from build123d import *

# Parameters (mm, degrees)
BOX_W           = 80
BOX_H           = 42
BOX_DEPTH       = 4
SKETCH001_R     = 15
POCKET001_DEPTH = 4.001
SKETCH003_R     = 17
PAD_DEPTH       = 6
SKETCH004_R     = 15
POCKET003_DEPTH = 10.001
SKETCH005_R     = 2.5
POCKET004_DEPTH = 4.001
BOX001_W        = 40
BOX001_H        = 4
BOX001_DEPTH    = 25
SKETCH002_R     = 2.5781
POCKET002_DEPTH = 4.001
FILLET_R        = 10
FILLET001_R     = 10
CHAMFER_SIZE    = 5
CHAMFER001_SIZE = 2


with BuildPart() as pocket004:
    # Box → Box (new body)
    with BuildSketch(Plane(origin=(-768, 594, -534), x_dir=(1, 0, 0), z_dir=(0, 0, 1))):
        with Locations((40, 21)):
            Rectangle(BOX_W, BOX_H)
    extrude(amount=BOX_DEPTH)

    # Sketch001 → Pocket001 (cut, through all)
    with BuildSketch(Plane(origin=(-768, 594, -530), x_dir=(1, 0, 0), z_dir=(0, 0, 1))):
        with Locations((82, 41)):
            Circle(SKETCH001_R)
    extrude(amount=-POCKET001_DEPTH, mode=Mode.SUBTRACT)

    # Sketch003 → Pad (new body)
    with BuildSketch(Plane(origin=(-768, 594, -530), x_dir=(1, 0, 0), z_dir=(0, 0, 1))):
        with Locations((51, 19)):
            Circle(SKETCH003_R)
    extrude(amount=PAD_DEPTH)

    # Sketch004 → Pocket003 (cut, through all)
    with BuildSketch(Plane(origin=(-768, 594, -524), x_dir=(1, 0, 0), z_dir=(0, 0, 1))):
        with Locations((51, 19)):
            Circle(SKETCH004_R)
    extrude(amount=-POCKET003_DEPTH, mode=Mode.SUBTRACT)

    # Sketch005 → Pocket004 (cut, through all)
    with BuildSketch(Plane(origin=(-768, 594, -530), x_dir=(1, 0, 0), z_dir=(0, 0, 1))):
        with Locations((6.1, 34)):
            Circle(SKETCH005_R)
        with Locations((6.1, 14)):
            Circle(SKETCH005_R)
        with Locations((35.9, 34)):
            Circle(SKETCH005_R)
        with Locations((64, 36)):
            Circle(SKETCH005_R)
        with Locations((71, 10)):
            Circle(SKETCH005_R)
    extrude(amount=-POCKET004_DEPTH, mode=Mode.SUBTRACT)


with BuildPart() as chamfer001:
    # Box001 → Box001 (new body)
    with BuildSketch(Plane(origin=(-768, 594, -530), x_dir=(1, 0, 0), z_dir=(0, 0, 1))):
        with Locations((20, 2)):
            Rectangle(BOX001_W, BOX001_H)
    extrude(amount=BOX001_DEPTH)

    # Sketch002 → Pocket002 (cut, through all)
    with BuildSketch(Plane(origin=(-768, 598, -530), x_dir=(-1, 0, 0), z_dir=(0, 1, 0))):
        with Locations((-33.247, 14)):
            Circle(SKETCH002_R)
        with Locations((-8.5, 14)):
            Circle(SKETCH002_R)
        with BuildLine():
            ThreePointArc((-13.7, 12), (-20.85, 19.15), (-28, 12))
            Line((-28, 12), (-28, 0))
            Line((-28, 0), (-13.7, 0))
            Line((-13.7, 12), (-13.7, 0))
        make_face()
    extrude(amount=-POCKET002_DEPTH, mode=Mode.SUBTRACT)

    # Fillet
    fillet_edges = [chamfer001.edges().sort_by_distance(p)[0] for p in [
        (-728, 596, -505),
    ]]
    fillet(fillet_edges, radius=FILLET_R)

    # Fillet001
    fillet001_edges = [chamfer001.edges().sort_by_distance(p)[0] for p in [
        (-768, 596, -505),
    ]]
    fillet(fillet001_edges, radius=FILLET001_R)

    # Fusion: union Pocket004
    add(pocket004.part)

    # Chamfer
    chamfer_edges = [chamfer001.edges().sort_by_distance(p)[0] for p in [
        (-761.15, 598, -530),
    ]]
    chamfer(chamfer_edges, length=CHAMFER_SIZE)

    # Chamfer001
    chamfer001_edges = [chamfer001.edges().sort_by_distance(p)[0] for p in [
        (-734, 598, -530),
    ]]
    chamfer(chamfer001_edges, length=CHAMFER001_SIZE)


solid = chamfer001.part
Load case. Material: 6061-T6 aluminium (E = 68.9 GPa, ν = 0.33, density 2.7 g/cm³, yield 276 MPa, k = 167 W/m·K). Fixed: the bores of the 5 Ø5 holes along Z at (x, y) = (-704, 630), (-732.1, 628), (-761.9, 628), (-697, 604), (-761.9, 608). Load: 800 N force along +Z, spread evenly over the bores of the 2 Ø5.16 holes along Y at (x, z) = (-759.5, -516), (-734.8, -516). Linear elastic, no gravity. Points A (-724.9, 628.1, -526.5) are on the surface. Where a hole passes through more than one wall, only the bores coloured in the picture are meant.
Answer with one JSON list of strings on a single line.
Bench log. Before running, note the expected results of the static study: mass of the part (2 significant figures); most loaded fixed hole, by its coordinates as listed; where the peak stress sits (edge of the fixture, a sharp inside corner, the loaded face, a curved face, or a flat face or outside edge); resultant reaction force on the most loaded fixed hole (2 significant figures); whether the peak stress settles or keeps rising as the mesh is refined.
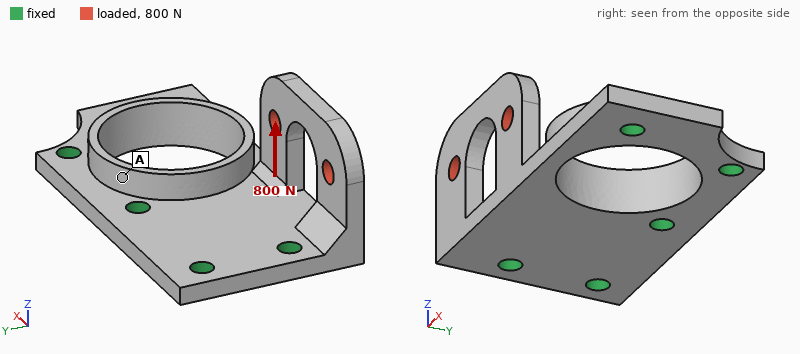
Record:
["37 g", "(-761.9, 608)", "edge of the fixture", "670 N", "keeps rising"]
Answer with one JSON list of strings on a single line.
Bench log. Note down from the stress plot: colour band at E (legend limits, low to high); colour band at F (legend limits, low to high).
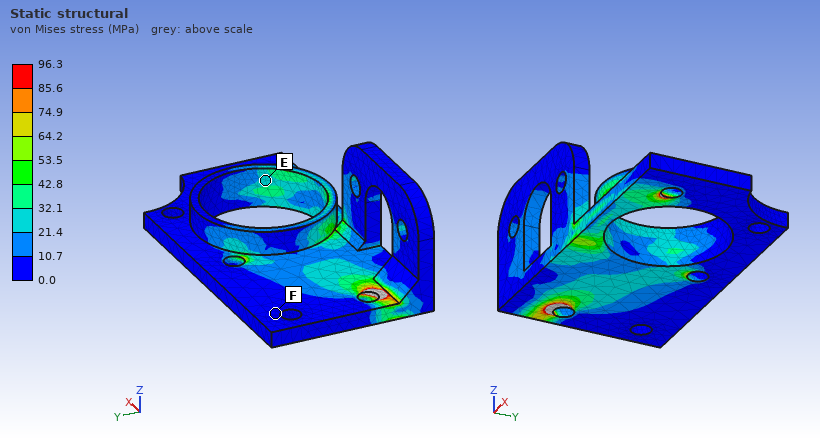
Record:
["21.4 to 32.1 MPa", "0.0 to 10.7 MPa"]
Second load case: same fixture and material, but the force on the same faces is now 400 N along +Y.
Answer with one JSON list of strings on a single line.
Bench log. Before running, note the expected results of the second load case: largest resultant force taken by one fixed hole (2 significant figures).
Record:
["200 N"]
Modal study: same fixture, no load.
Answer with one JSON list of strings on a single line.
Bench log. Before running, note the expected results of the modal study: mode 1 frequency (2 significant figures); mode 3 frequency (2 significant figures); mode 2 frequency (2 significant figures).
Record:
["3200 Hz", "7200 Hz", "5000 Hz"]
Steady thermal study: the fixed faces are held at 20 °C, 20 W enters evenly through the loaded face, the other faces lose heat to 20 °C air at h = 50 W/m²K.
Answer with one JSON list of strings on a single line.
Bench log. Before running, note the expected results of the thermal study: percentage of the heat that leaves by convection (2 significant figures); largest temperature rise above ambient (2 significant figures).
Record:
["14 %", "29 K"]
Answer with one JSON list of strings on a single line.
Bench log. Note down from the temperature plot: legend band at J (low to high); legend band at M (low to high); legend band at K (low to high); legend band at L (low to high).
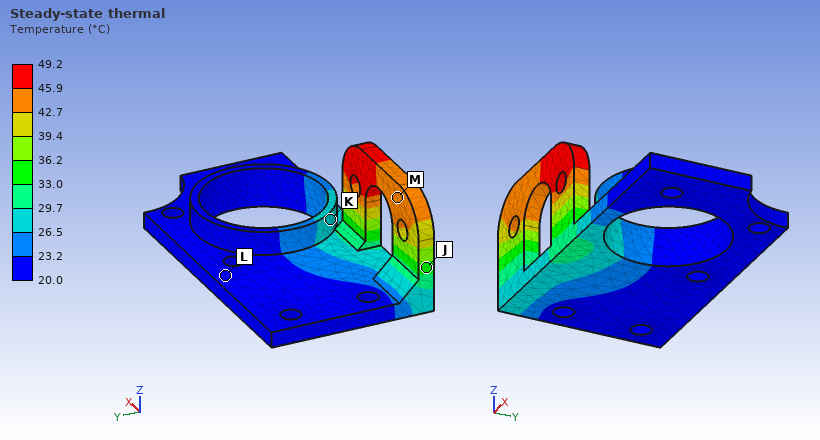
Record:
["33.0 to 36.2 °C", "42.7 to 45.9 °C", "26.5 to 29.7 °C", "20.0 to 23.2 °C"]
